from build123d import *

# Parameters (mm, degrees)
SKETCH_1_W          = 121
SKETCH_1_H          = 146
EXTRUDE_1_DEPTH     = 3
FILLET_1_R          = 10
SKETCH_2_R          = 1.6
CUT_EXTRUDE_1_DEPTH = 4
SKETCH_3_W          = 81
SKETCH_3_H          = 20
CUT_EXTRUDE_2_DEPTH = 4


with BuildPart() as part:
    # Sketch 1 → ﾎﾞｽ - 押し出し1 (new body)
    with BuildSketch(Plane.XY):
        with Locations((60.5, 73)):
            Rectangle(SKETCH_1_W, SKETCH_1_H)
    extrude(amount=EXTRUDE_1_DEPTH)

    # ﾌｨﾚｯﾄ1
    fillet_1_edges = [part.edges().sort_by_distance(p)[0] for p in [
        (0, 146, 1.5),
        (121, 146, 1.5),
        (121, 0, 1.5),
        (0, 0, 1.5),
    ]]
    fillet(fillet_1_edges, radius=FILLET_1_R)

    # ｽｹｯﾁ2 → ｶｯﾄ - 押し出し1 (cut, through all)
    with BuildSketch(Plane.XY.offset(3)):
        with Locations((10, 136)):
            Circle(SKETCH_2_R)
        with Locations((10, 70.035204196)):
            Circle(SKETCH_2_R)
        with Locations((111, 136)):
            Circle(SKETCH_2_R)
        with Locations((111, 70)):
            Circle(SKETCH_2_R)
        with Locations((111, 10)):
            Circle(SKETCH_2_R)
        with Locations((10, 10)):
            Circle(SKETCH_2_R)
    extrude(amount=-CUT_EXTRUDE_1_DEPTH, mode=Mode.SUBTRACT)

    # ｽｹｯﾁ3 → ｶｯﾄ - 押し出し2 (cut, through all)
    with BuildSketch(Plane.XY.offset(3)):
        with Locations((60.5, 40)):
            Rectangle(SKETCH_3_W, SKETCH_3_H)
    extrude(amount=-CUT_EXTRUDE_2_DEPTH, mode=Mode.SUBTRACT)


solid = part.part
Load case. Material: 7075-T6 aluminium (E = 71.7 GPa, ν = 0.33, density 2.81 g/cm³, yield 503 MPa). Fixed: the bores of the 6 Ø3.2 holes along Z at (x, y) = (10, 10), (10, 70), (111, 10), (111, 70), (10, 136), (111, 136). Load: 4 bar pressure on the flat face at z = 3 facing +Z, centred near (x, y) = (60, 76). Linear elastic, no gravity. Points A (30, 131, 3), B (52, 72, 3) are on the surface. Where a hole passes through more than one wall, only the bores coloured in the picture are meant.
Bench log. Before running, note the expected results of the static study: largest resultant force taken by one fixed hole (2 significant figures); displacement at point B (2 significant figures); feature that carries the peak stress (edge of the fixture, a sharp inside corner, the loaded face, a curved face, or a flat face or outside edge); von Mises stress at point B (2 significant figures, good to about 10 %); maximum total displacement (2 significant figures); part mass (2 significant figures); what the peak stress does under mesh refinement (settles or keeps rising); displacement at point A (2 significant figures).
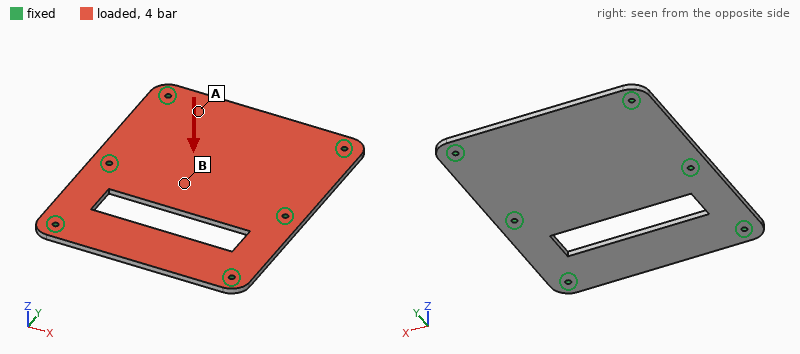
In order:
1.4 kN
0.91 mm
edge of the fixture
120 MPa
1.0 mm
130 g
keeps rising
0.45 mm
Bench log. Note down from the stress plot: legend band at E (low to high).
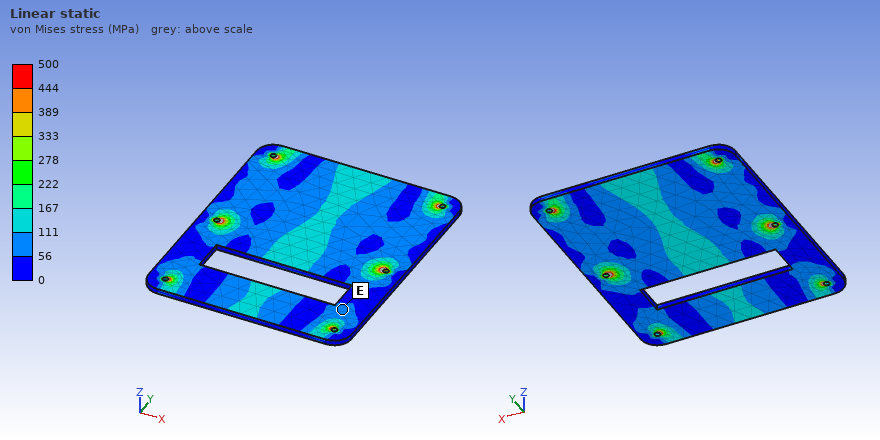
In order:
56 to 111 MPa
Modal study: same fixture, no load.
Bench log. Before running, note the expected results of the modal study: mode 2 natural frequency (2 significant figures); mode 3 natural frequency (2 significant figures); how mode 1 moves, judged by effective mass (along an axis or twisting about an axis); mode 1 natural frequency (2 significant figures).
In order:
1400 Hz
1800 Hz
along Z
1300 Hz
